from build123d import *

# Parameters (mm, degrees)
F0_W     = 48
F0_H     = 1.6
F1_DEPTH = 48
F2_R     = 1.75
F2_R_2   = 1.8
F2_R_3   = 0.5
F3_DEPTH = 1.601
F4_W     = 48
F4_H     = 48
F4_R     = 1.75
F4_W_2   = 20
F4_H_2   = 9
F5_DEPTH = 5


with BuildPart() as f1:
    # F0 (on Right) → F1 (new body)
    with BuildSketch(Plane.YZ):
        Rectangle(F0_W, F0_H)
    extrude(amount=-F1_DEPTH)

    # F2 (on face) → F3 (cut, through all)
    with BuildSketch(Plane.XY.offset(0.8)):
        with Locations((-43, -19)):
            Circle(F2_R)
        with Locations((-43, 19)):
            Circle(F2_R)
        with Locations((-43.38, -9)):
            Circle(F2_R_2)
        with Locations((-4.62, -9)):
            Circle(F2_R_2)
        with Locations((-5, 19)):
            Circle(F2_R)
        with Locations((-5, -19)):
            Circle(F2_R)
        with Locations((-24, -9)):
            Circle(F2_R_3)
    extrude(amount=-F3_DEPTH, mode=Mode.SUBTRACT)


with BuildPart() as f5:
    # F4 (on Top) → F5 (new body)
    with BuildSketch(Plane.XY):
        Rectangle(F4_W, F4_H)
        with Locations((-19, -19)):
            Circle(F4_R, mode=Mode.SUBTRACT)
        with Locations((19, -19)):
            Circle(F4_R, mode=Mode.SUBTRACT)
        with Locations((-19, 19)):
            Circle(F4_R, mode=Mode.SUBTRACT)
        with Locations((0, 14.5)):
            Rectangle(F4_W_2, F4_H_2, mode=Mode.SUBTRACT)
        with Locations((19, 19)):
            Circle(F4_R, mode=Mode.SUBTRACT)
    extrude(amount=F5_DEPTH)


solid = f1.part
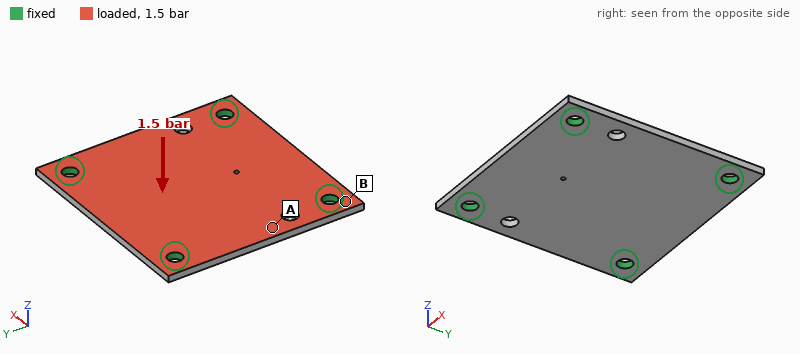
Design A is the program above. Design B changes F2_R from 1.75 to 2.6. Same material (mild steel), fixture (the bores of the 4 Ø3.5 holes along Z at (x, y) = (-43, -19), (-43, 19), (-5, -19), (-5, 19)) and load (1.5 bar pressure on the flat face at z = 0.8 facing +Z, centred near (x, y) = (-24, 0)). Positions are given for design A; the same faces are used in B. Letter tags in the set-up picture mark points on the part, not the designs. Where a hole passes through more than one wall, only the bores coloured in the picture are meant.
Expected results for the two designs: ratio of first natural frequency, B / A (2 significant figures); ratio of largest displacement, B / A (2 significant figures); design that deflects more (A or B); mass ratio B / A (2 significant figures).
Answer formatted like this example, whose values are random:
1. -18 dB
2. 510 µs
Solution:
1. 1.1
2. 0.83
3. A
4. 0.98
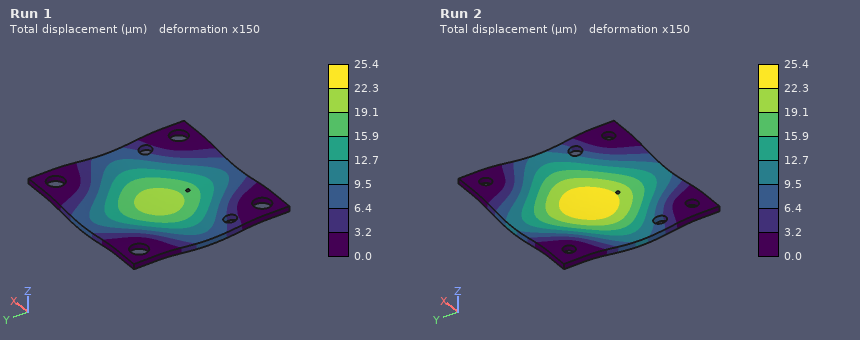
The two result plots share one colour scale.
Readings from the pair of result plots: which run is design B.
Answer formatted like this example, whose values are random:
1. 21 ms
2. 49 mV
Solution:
1. Run 1
